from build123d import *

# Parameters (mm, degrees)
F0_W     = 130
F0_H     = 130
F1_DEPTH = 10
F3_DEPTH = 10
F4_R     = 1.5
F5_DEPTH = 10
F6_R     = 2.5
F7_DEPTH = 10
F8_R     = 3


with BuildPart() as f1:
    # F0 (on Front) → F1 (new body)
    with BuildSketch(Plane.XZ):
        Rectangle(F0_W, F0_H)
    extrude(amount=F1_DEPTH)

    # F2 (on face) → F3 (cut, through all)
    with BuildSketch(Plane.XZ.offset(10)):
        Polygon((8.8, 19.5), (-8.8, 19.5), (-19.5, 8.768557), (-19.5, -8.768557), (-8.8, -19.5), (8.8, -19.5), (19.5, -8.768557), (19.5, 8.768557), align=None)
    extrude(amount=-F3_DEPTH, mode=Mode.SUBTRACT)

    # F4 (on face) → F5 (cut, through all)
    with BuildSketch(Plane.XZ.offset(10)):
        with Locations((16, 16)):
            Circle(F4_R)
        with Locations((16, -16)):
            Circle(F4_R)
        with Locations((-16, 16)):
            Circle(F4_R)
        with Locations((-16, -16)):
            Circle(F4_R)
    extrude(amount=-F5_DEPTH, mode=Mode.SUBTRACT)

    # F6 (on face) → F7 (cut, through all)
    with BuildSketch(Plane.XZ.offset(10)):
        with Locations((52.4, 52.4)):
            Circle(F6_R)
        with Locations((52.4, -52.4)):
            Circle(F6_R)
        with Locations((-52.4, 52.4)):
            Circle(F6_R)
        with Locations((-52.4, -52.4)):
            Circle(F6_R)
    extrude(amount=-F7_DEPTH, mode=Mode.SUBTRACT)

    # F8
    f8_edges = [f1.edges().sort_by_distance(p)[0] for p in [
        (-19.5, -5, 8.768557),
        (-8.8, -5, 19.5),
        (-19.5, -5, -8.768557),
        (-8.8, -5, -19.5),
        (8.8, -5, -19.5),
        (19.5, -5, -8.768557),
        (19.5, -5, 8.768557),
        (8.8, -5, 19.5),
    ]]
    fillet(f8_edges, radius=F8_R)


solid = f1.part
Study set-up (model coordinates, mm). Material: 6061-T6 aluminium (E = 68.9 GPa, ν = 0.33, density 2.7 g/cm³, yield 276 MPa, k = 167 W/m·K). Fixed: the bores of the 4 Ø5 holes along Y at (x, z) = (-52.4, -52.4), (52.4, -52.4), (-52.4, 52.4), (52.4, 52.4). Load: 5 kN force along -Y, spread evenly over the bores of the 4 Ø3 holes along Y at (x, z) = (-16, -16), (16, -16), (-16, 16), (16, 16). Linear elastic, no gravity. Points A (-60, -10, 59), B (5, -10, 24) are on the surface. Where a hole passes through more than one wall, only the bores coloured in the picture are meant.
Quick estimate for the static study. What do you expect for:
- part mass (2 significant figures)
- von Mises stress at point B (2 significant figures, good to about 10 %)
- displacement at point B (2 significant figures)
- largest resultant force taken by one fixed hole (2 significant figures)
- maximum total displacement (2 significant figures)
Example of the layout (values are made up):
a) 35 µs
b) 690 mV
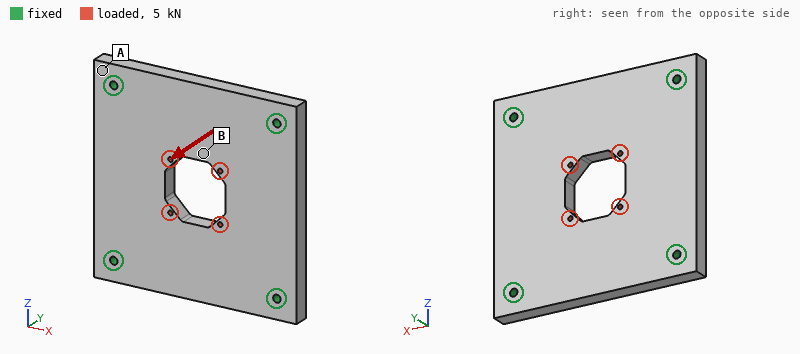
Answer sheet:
a) 420 g
b) 42 MPa
c) 0.14 mm
d) 1.3 kN
e) 0.16 mm
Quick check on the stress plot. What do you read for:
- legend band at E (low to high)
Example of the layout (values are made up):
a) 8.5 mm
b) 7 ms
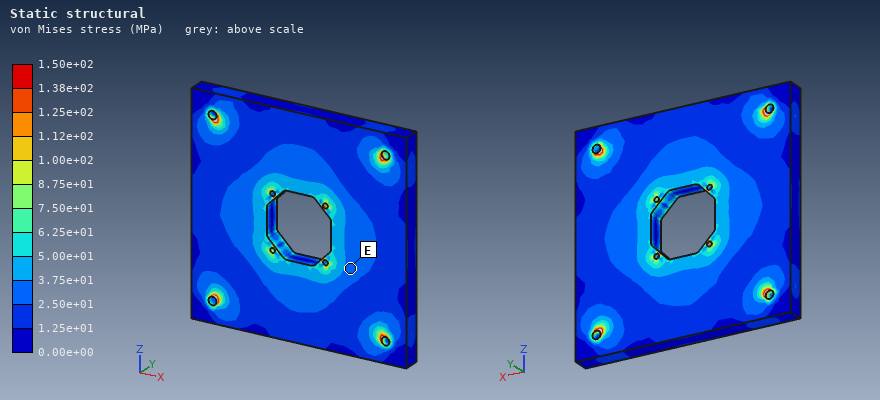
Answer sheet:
a) 2.50e+01 to 3.75e+01 MPa
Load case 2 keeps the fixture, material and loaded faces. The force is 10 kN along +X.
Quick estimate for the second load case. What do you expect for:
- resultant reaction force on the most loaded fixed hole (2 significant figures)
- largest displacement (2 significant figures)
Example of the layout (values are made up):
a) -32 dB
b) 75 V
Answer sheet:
a) 2.7 kN
b) 13 µm
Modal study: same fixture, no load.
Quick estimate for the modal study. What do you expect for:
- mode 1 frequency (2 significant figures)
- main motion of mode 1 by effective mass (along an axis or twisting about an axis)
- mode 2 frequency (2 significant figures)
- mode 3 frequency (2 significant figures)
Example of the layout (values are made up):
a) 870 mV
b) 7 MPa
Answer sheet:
a) 2900 Hz
b) along Y
c) 4500 Hz
d) 4500 Hz
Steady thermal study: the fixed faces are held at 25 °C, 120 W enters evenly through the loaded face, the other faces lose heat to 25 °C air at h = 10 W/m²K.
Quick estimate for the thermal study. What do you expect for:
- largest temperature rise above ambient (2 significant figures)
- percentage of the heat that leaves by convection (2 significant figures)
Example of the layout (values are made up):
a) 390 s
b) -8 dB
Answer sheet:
a) 29 K
b) 3.6 %
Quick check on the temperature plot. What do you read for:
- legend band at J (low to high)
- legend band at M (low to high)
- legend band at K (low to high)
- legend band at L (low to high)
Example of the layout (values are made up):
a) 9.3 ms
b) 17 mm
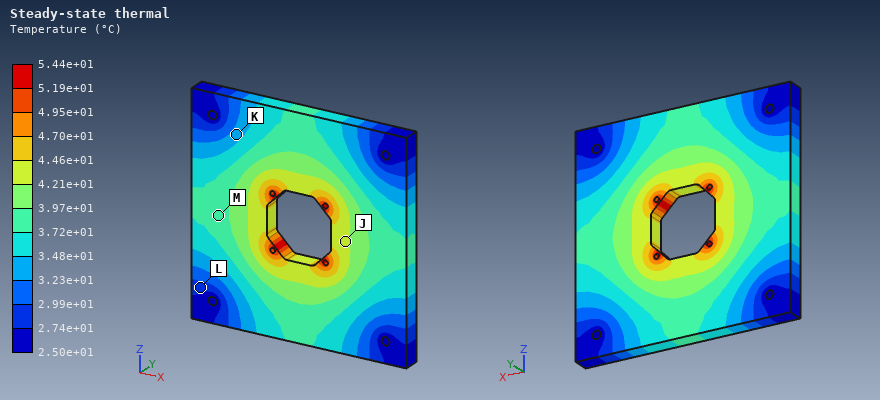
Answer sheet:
a) 4.21e+01 to 4.46e+01 °C
b) 3.72e+01 to 3.97e+01 °C
c) 3.23e+01 to 3.48e+01 °C
d) 2.74e+01 to 2.99e+01 °C
